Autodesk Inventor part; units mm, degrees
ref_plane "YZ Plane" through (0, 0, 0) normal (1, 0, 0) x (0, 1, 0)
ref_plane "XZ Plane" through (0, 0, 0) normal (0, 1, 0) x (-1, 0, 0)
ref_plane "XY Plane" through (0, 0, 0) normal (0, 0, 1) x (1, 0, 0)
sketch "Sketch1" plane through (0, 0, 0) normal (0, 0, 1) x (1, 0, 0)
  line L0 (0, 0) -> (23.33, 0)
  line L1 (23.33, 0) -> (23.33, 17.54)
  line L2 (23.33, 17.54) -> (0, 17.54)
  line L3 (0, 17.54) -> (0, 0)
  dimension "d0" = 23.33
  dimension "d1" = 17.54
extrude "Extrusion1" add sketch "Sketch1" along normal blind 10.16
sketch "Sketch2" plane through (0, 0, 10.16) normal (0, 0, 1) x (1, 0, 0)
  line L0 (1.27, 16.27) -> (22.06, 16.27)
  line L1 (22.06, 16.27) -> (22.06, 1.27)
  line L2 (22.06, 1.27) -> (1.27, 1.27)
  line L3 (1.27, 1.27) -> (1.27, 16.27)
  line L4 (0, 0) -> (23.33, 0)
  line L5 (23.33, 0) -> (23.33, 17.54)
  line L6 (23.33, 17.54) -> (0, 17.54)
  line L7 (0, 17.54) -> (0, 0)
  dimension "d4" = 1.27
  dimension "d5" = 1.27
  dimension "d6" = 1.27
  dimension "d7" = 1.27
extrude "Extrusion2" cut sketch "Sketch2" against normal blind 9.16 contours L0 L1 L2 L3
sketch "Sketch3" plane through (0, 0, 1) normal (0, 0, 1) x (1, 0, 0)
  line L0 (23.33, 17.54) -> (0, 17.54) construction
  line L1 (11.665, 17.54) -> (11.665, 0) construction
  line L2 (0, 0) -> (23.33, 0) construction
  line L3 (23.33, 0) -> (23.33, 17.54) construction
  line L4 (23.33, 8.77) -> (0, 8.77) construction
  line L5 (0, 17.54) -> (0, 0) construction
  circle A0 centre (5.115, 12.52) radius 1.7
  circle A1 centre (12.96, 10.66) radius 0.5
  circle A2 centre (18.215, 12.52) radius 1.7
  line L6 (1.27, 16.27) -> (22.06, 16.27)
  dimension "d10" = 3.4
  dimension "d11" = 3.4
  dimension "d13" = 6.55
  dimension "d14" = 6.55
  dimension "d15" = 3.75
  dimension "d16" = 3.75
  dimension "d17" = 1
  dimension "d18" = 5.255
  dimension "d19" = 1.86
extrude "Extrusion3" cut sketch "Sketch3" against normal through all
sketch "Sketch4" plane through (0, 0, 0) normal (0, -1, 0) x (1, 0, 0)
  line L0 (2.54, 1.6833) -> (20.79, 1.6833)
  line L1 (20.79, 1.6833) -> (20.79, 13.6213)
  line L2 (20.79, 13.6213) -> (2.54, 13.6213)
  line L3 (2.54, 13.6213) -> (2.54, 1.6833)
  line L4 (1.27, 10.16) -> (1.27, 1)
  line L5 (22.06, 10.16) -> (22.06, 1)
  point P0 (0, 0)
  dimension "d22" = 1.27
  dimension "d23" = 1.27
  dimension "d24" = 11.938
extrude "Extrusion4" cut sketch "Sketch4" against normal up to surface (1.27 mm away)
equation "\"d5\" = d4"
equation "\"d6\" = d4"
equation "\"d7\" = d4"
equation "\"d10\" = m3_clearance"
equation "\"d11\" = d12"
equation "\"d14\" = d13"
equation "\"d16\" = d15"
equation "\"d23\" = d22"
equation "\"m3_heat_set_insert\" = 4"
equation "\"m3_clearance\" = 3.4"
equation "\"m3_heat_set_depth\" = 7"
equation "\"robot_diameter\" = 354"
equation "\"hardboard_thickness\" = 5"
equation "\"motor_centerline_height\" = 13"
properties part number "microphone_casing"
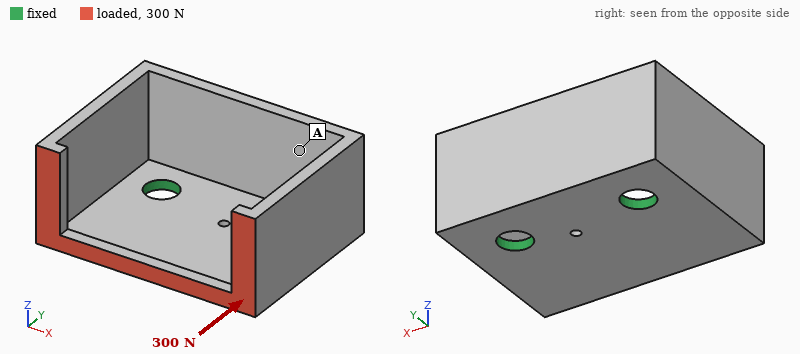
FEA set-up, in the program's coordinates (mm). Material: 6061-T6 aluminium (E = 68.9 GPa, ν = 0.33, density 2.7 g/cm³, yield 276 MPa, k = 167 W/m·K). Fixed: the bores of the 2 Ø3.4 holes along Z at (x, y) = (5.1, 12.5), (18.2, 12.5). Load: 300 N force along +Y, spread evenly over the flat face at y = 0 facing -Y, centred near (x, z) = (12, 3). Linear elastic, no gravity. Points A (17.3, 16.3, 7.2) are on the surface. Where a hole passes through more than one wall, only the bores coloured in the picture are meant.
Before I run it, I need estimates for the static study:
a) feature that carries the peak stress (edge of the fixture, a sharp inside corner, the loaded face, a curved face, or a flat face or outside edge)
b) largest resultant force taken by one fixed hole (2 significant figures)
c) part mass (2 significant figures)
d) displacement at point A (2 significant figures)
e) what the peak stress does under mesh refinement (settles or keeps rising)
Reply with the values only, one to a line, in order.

edge of the fixture
150 N
2.9 g
34 µm
keeps rising
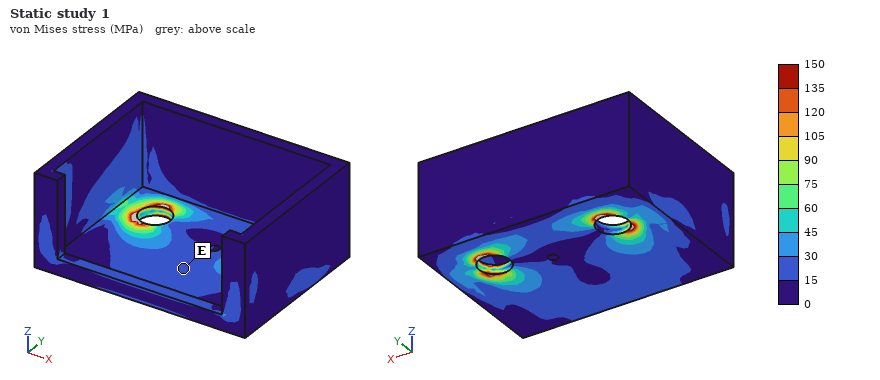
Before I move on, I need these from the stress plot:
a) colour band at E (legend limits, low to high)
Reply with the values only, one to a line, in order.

15 to 30 MPa
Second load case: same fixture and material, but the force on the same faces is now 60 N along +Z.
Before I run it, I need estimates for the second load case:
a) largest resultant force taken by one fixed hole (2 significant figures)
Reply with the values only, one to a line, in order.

30 N
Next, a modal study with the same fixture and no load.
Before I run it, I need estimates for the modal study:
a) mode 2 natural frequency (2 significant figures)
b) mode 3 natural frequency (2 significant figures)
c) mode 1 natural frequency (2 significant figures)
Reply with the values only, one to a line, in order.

6600 Hz
8600 Hz
5400 Hz
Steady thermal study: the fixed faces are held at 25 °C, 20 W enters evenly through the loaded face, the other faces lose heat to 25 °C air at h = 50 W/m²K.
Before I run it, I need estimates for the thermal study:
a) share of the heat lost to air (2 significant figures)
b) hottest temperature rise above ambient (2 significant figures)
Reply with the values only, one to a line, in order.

7.8 %
41 K
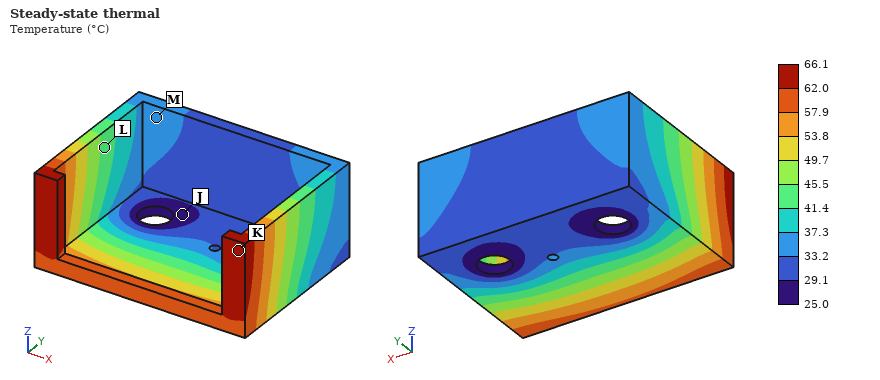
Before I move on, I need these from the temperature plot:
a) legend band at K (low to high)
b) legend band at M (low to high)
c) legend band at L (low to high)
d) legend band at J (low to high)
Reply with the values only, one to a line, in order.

62.0 to 66.1 °C
33.2 to 37.3 °C
41.4 to 45.5 °C
25.0 to 29.1 °C
